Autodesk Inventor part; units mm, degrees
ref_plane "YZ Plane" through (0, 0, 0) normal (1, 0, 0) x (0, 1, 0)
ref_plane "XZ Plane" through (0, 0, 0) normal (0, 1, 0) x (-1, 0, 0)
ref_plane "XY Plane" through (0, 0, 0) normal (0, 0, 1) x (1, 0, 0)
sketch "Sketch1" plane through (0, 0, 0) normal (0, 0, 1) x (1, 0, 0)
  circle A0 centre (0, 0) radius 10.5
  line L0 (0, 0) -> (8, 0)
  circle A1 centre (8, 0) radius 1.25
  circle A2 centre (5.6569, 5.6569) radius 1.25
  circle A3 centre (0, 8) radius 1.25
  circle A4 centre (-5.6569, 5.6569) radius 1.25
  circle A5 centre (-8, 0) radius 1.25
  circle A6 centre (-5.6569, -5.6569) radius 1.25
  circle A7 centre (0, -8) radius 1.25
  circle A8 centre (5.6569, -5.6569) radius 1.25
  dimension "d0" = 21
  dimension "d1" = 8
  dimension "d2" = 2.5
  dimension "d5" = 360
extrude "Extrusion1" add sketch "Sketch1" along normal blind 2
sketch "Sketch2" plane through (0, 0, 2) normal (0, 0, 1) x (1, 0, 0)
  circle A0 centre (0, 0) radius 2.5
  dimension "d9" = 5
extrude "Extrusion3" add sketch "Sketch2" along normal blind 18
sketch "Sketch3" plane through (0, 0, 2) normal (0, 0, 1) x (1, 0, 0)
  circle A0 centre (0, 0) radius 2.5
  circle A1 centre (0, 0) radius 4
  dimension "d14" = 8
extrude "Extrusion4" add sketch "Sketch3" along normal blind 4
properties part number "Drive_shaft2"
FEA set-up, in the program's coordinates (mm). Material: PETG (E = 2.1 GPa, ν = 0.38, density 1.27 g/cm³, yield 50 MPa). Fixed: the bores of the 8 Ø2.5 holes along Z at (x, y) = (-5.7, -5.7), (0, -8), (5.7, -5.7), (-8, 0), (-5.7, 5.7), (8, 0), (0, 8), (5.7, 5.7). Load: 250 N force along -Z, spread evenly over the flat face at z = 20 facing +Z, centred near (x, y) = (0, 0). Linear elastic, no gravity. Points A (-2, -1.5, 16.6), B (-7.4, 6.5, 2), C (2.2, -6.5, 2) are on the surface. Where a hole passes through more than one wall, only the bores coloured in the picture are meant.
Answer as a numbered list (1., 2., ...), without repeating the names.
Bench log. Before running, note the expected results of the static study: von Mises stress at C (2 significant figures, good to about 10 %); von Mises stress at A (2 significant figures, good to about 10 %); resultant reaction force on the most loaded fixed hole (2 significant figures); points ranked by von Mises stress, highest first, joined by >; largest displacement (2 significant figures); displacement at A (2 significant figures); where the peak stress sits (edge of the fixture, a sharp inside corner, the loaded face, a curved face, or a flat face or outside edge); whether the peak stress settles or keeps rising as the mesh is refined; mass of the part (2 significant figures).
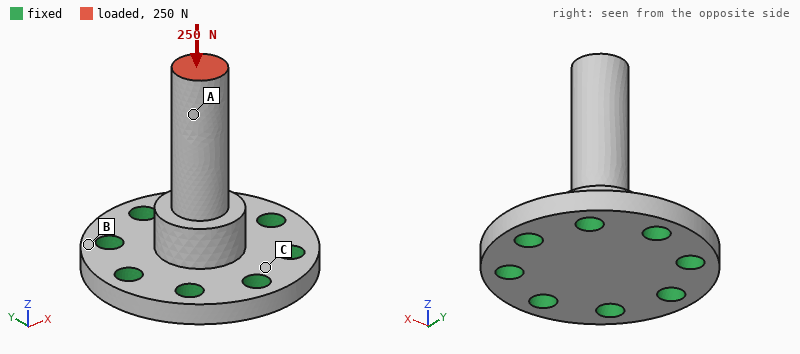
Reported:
1. 6.1 MPa
2. 13 MPa
3. 35 N
4. A > C > B
5. 0.15 mm
6. 0.13 mm
7. edge of the fixture
8. keeps rising
9. 1.4 g
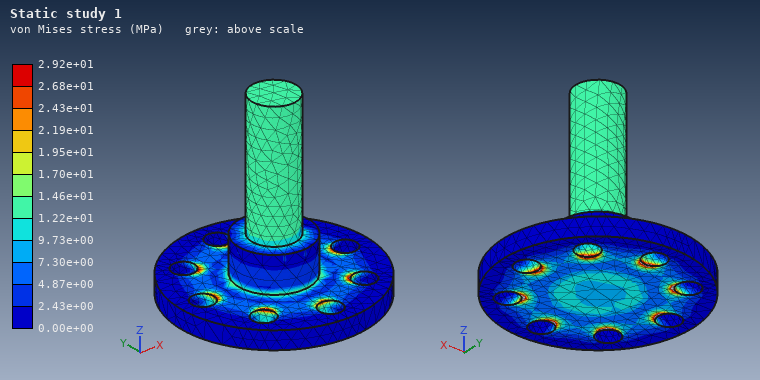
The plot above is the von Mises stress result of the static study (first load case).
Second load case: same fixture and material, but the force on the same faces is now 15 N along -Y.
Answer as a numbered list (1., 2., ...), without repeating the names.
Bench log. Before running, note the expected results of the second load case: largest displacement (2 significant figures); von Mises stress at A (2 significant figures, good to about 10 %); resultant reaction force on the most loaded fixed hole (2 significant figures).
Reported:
1. 0.37 mm
2. 2.9 MPa
3. 13 N
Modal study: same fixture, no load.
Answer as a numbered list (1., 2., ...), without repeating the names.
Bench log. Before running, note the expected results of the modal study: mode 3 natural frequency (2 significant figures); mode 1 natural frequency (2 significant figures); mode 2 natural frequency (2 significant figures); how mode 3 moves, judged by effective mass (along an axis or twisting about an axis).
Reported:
1. 11 kHz
2. 3100 Hz
3. 3100 Hz
4. along Z
